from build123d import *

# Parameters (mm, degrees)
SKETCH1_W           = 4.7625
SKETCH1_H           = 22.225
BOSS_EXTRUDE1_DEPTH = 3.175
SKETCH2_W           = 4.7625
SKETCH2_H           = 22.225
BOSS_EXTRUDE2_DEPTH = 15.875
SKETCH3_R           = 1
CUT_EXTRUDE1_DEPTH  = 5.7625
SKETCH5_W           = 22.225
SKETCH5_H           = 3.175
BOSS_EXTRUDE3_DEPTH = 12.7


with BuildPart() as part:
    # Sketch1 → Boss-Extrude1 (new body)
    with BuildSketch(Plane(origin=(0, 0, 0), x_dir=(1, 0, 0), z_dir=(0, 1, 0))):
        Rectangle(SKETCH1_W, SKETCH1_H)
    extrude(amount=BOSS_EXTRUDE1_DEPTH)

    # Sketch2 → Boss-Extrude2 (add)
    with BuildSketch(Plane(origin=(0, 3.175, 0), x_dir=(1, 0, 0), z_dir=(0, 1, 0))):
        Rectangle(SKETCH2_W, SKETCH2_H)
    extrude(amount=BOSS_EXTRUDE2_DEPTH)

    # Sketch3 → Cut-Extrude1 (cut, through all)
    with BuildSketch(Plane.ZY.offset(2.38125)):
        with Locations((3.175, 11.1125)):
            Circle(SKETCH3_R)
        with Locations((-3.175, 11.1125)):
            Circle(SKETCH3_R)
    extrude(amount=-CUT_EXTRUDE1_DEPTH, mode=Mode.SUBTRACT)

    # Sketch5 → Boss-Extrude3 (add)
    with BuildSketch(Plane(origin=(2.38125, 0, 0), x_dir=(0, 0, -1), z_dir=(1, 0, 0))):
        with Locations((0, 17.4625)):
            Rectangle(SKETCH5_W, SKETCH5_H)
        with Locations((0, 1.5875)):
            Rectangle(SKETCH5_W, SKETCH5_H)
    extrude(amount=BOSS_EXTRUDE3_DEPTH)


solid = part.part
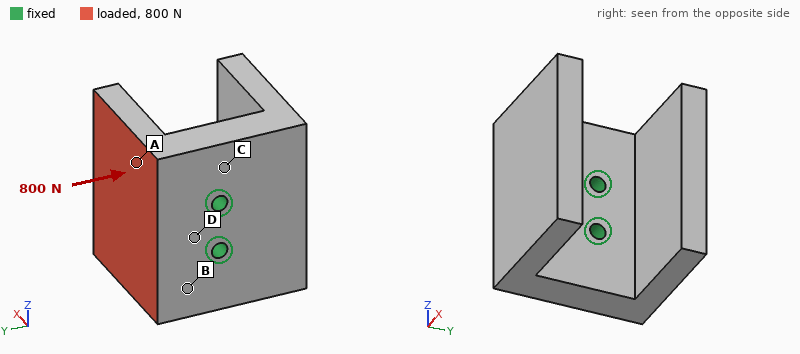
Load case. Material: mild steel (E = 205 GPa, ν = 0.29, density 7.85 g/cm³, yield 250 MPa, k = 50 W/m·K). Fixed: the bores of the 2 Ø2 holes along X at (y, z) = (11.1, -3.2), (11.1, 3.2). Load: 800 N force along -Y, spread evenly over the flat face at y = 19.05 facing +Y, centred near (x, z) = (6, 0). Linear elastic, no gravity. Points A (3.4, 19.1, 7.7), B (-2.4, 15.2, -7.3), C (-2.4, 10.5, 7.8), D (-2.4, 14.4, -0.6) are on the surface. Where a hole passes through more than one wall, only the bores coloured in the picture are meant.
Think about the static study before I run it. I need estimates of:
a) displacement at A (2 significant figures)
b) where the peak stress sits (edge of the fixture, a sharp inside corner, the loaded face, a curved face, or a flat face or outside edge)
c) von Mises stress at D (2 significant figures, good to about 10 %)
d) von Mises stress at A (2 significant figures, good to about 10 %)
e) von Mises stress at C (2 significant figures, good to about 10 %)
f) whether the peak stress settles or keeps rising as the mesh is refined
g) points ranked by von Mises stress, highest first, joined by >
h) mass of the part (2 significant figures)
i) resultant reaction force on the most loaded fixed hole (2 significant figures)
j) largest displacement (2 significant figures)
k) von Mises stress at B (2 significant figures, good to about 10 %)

7.2 µm
edge of the fixture
51 MPa
72 MPa
21 MPa
keeps rising
A > D > B > C
30 g
400 N
32 µm
38 MPa
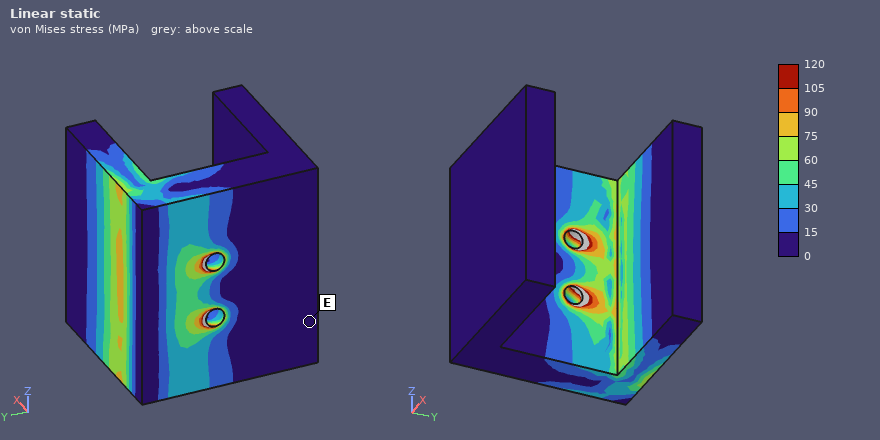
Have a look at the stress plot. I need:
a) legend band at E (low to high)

0 to 15 MPa
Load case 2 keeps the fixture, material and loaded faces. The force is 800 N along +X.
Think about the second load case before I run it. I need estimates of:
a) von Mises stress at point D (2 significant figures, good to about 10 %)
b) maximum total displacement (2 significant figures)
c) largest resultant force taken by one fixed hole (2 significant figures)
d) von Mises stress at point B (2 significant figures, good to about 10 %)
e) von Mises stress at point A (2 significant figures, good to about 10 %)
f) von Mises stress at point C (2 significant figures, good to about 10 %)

44 MPa
18 µm
400 N
26 MPa
27 MPa
25 MPa
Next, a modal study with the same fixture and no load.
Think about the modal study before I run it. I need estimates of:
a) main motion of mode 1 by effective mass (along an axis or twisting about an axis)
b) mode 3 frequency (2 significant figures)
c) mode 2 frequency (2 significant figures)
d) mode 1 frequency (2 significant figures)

along Y
12 kHz
10 kHz
8400 Hz
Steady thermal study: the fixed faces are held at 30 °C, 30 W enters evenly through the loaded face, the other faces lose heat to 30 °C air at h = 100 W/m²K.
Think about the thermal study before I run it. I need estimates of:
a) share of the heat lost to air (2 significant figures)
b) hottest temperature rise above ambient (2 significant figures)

15 %
77 K
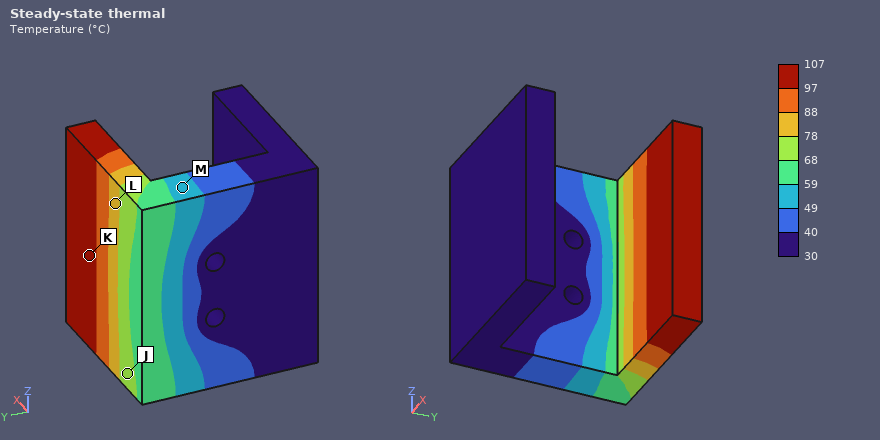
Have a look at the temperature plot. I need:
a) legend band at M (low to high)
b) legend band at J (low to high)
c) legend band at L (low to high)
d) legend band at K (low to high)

49 to 59 °C
68 to 78 °C
78 to 88 °C
97 to 107 °C
